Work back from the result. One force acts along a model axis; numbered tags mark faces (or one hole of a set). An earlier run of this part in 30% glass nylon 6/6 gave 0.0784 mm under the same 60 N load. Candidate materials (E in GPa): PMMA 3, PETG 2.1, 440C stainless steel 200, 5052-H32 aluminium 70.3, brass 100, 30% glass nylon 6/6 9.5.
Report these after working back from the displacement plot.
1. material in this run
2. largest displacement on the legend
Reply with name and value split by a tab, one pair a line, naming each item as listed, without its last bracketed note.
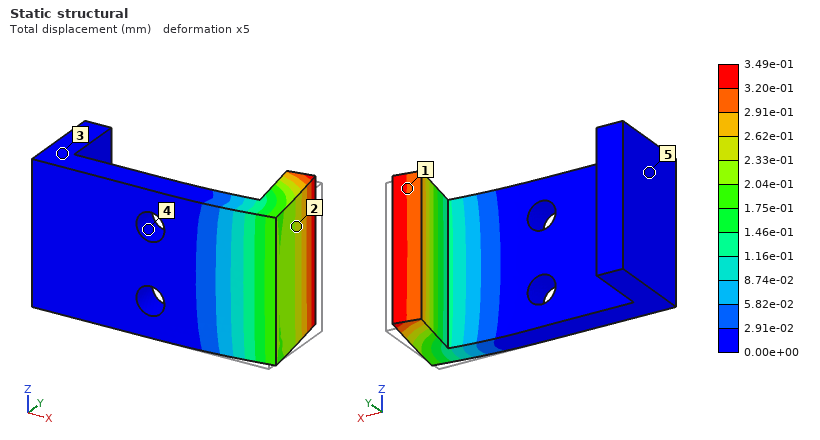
material in this run	PETG
largest displacement on the legend	3.49e-01 mm
